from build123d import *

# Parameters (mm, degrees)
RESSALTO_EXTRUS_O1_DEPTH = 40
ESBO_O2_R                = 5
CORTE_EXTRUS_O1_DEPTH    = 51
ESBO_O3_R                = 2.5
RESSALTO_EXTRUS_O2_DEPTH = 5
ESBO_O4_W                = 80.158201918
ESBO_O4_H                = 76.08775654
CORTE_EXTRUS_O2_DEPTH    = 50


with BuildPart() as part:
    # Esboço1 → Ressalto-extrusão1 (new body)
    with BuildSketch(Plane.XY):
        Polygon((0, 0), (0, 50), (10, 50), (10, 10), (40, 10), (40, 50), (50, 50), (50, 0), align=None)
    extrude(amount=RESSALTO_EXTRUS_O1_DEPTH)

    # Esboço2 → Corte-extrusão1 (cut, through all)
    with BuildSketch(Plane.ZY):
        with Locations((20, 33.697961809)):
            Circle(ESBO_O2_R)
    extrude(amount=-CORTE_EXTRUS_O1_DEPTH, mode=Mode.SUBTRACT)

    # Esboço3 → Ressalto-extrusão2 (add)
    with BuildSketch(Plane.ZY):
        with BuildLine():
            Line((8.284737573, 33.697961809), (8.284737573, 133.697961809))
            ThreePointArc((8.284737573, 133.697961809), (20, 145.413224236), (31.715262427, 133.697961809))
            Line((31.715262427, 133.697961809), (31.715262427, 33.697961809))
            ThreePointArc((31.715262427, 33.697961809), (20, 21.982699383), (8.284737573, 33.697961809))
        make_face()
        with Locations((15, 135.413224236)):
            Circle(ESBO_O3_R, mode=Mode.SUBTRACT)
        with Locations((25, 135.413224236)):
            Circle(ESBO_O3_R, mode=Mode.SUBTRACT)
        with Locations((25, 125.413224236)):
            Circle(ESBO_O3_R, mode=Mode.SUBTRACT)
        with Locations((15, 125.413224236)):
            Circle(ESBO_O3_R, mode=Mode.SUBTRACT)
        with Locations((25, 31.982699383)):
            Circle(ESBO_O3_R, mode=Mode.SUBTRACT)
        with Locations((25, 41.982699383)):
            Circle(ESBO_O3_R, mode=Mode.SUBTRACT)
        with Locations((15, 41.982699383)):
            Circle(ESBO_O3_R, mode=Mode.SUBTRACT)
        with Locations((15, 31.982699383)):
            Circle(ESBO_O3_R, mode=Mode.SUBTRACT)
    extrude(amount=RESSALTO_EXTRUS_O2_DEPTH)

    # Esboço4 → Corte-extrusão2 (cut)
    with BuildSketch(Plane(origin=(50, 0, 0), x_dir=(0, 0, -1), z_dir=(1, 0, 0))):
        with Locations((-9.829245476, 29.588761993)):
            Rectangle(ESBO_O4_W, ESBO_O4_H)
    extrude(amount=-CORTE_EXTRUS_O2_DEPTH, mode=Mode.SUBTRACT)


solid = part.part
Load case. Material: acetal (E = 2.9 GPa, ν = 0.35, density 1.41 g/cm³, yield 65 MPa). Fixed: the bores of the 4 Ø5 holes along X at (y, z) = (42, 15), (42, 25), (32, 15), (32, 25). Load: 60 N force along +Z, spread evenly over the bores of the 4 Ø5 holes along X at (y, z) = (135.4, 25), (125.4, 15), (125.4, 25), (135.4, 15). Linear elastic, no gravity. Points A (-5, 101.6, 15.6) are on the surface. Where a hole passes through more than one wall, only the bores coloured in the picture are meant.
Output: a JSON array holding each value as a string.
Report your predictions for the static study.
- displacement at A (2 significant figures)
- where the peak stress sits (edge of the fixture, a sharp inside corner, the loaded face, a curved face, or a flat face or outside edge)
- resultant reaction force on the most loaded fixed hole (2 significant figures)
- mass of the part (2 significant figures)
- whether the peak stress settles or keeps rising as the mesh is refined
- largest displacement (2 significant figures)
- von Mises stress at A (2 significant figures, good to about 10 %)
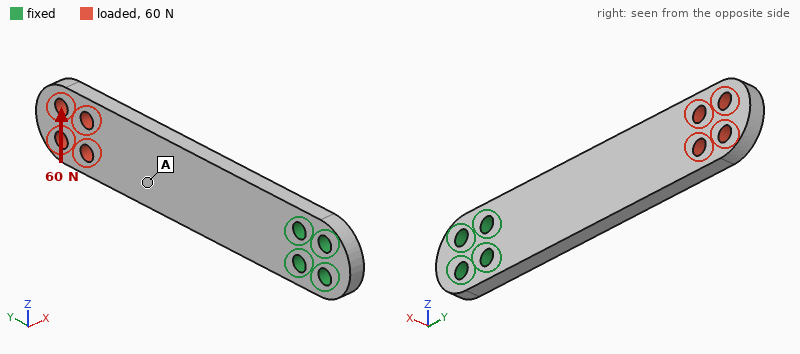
["0.53 mm", "edge of the fixture", "320 N", "18 g", "keeps rising", "1.2 mm", "1.8 MPa"]
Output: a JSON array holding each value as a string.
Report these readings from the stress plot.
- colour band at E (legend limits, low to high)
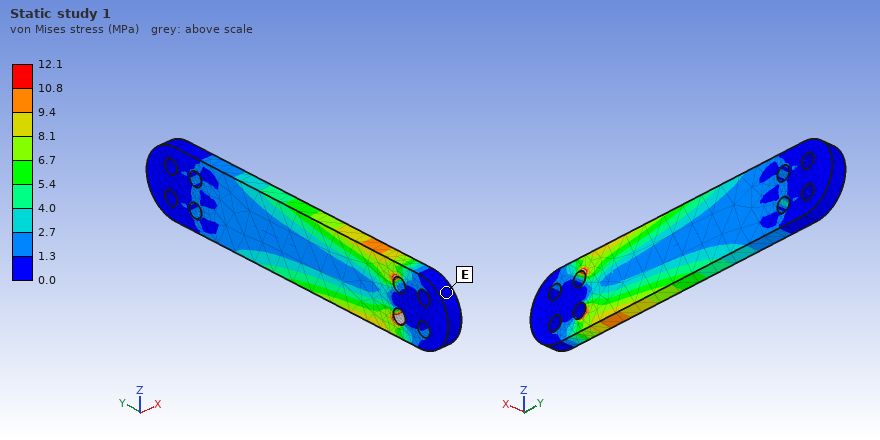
["0.0 to 1.3 MPa"]
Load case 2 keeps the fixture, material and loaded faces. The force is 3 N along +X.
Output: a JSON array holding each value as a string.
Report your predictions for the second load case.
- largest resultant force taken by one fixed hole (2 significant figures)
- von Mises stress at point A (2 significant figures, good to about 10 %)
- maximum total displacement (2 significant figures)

["2.8 N", "0.89 MPa", "1.2 mm"]
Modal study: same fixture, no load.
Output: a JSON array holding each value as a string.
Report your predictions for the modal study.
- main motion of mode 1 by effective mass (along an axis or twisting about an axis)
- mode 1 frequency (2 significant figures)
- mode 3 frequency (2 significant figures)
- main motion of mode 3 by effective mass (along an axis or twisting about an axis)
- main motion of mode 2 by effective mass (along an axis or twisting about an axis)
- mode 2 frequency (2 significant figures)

["along X", "120 Hz", "730 Hz", "along X", "along Z", "530 Hz"]
